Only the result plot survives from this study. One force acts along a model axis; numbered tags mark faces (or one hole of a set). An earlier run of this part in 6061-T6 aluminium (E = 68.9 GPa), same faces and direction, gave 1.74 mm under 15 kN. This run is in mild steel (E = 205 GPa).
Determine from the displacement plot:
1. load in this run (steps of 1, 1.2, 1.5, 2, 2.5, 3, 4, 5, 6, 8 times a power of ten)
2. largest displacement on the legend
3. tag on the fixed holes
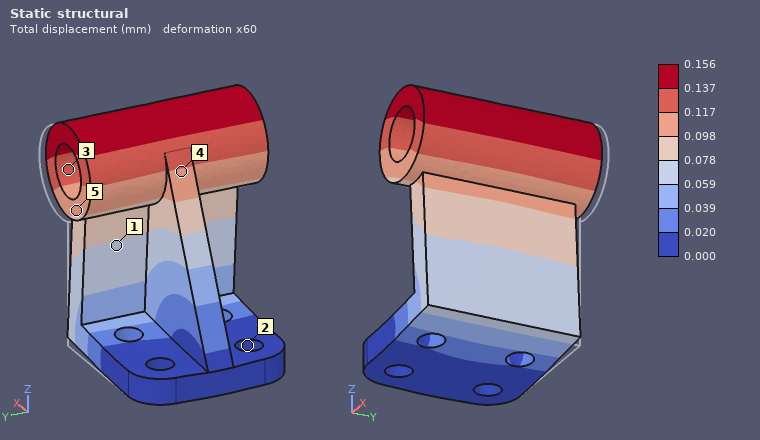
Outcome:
4 kN
0.156 mm
2
